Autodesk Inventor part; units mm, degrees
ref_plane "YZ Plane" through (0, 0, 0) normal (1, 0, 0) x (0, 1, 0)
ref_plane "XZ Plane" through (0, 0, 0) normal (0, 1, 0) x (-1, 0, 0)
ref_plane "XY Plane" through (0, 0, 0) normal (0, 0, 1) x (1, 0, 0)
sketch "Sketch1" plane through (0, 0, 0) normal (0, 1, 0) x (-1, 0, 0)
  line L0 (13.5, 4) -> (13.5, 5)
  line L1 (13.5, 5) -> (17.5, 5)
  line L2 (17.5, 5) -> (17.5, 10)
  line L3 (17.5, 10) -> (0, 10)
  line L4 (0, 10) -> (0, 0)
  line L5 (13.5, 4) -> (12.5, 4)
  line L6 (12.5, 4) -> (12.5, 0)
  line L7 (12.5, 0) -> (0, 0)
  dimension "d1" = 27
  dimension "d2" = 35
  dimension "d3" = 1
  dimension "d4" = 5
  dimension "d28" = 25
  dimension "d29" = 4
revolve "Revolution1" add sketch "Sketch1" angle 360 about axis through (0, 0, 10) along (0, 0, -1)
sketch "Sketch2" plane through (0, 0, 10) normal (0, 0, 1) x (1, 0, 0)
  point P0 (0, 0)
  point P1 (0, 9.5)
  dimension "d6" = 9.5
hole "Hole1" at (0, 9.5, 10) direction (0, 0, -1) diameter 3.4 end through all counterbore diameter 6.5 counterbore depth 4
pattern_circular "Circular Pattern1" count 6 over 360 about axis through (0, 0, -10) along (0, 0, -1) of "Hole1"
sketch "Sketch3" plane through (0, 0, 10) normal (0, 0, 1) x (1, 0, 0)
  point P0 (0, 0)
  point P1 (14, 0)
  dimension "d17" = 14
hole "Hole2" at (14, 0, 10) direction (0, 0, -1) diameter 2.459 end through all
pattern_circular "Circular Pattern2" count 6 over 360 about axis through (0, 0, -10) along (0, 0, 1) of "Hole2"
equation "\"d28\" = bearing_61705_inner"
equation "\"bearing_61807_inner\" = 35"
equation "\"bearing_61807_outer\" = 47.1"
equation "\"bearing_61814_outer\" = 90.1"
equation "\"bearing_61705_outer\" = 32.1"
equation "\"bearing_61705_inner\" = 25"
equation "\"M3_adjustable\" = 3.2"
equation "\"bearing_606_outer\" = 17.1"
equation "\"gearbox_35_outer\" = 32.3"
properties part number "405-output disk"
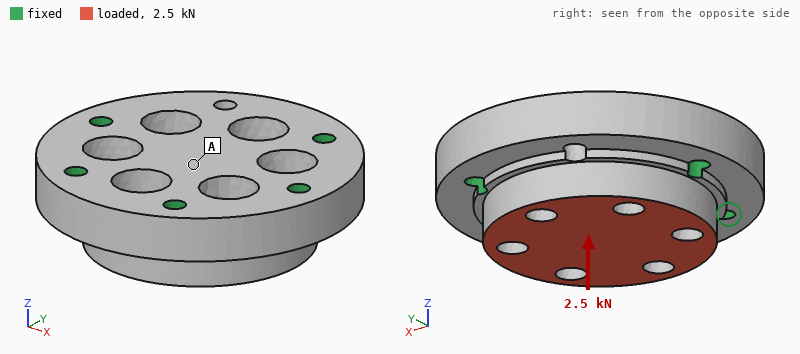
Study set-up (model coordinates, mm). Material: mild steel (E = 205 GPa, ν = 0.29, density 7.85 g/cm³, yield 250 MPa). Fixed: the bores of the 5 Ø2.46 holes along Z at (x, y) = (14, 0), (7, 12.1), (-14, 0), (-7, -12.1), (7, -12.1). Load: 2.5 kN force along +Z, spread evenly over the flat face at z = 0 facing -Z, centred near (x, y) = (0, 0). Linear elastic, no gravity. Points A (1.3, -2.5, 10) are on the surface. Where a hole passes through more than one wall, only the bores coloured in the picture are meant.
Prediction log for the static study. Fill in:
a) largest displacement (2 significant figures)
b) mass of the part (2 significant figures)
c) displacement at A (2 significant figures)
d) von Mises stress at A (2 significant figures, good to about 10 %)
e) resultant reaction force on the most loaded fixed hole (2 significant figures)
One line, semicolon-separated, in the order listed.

2.1 µm; 48 g; 1.2 µm; 7.4 MPa; 720 N
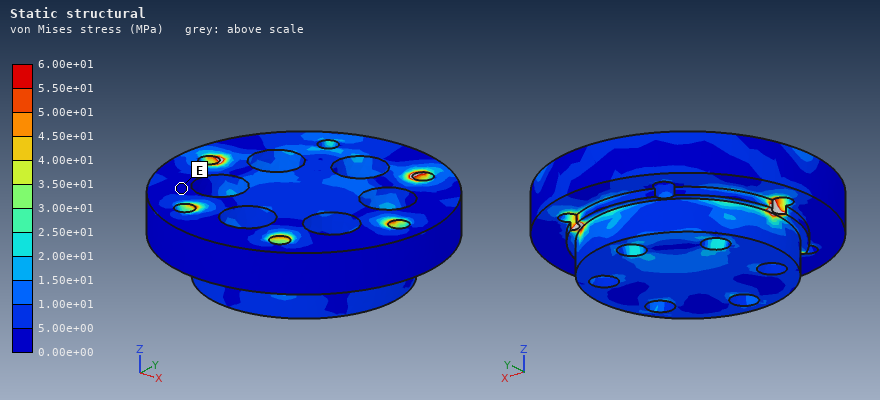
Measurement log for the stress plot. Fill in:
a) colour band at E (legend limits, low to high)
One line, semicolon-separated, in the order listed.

0.00e+00 to 5.00e+00 MPa
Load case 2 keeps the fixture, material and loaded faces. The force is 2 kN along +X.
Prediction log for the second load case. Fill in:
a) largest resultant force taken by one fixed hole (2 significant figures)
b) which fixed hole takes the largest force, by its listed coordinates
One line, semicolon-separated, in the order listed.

690 N; (-14, 0)
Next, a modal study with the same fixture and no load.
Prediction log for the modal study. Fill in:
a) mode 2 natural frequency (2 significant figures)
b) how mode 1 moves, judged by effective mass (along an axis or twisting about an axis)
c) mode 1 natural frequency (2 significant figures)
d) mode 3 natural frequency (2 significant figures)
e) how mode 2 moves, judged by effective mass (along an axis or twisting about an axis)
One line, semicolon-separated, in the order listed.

48 kHz; along Z; 30 kHz; 54 kHz; along Z
